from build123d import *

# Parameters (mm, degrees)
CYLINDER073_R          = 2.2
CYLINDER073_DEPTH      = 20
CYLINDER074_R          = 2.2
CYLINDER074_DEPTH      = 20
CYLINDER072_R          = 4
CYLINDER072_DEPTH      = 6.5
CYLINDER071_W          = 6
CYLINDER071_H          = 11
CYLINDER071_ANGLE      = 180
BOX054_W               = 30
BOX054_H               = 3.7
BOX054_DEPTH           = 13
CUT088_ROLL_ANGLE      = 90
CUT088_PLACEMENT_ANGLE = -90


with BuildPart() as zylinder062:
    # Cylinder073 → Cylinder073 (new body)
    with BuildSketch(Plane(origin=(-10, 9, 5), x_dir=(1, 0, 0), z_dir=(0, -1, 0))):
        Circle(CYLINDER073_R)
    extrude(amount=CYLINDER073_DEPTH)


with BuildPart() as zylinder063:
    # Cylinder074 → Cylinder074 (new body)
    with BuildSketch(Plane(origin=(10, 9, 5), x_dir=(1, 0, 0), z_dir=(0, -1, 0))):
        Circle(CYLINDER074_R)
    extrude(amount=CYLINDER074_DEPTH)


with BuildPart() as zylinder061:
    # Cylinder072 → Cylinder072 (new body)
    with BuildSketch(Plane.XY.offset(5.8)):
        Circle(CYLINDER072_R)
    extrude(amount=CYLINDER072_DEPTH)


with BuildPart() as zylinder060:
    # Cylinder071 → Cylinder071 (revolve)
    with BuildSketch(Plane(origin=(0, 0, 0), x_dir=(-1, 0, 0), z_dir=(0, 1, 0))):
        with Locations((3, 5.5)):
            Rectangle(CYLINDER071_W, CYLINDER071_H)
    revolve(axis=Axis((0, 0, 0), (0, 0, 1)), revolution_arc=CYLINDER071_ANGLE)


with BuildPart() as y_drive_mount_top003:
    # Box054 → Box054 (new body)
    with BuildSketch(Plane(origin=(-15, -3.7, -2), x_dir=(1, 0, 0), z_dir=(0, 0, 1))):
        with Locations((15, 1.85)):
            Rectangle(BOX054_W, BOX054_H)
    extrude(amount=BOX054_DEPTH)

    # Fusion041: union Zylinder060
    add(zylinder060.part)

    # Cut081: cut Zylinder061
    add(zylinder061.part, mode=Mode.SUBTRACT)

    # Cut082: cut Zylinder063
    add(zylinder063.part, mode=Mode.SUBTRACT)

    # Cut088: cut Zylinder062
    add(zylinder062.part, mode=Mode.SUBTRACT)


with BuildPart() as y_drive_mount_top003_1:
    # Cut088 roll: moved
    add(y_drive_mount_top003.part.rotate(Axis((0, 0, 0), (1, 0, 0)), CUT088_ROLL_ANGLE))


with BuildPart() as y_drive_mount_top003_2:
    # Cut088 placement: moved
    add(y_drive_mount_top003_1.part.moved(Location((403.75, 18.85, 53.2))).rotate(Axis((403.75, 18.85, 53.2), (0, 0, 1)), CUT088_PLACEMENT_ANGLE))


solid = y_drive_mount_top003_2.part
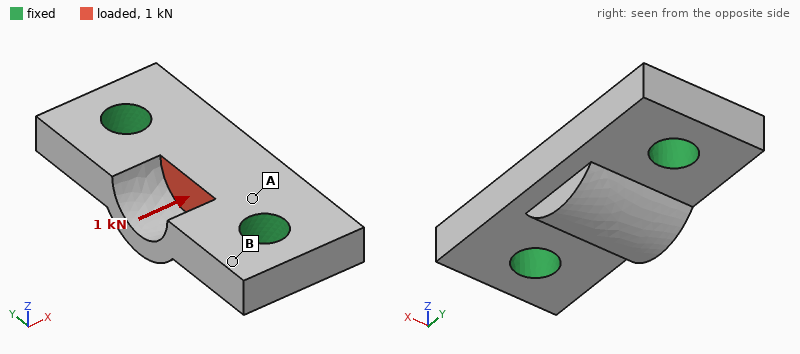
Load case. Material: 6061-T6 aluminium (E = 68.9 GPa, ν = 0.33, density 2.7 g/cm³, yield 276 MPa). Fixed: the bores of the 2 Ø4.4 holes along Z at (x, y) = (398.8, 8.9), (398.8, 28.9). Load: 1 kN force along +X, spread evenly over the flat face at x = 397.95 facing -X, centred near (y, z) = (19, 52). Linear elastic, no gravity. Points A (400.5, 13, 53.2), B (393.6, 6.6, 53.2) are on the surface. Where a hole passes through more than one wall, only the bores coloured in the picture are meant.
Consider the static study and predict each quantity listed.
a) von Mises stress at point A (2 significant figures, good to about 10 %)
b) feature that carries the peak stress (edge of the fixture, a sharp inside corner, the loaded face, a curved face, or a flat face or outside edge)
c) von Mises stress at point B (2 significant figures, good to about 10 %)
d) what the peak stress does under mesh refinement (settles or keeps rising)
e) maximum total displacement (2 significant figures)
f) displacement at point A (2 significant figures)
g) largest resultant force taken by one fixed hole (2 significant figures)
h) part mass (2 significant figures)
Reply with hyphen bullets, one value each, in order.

- 31 MPa
- edge of the fixture
- 5.0 MPa
- keeps rising
- 7.7 µm
- 2.3 µm
- 530 N
- 3.7 g
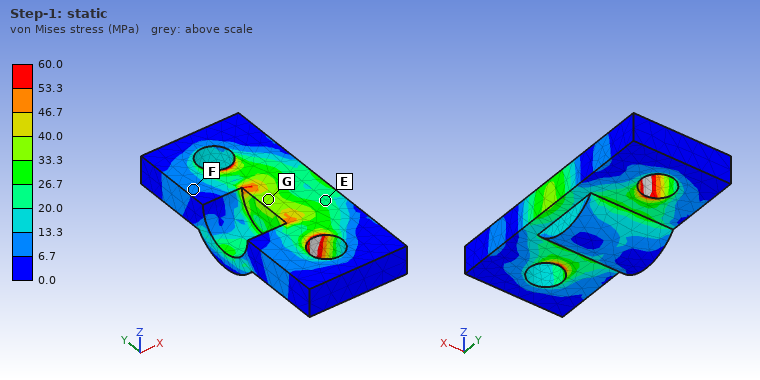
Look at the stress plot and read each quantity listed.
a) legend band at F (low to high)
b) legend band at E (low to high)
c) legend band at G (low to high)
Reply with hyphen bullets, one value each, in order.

- 6.7 to 13.3 MPa
- 20.0 to 26.7 MPa
- 33.3 to 40.0 MPa
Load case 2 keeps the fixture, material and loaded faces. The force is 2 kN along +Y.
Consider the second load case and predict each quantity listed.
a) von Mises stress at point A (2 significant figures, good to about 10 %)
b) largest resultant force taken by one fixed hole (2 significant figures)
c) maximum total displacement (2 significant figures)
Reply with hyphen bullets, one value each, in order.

- 45 MPa
- 1.0 kN
- 9.2 µm
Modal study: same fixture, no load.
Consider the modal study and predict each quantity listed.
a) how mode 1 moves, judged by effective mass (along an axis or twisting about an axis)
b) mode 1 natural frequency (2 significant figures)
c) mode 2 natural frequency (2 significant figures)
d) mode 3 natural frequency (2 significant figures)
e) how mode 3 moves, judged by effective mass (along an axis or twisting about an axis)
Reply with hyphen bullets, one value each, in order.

- along Z
- 41 kHz
- 51 kHz
- 66 kHz
- along X
